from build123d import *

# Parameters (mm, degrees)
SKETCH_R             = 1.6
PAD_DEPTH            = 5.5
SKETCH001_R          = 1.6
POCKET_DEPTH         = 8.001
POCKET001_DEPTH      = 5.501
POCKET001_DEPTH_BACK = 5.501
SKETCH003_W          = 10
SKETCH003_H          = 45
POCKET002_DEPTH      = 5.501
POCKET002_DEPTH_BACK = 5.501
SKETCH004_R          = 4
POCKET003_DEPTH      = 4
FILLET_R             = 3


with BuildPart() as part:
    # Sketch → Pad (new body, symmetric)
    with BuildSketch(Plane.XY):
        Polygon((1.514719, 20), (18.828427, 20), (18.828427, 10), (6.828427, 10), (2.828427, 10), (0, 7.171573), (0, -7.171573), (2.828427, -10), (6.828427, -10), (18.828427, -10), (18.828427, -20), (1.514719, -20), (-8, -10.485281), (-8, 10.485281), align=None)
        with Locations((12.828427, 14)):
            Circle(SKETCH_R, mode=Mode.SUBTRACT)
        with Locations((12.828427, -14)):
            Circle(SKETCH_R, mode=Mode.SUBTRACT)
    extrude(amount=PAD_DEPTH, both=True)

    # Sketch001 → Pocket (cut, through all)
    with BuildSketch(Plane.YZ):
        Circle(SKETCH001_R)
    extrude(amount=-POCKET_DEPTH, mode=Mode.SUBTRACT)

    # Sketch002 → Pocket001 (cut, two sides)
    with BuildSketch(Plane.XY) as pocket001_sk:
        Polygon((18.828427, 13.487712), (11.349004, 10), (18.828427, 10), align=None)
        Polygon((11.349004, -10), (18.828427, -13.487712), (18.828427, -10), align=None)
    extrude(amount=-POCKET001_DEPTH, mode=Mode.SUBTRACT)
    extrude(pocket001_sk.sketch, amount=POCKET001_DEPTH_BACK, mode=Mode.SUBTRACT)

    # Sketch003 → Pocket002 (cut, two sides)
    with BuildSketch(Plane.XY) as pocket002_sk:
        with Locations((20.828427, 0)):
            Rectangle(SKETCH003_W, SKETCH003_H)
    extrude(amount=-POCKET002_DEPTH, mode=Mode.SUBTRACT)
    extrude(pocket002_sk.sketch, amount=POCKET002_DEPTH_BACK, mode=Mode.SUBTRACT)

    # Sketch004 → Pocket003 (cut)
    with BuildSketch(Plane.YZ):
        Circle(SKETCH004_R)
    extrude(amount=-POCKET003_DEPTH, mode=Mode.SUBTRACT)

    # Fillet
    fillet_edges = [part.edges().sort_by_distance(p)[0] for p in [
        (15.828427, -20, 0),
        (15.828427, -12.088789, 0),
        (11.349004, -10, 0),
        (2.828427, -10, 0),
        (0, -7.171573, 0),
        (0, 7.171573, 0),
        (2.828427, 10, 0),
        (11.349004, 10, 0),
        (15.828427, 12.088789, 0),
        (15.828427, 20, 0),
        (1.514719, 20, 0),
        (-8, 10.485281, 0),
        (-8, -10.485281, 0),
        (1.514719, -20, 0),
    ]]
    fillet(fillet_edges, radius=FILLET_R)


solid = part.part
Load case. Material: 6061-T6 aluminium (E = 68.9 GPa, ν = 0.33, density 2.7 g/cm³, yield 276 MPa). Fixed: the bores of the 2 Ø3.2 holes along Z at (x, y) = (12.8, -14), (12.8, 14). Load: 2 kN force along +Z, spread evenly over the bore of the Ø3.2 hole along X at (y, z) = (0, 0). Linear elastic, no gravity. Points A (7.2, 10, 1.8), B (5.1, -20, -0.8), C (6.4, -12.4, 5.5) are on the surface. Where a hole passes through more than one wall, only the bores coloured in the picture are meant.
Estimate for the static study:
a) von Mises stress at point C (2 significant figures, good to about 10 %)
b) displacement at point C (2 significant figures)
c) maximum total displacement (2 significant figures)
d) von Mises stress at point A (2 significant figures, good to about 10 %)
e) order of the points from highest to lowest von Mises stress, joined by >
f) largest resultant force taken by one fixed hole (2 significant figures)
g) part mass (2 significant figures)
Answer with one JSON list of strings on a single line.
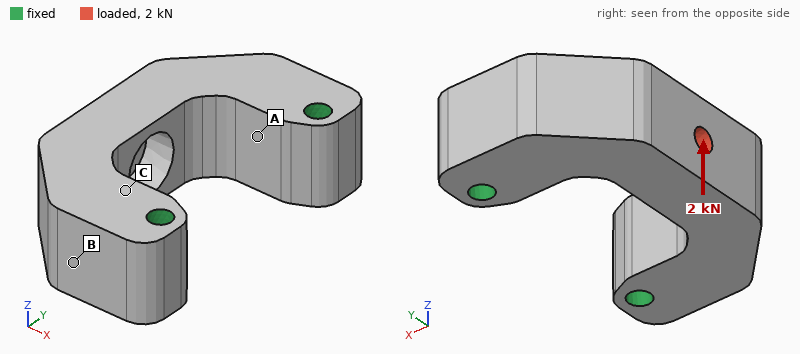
["85 MPa", "13 µm", "68 µm", "58 MPa", "C > A > B", "1.0 kN", "15 g"]
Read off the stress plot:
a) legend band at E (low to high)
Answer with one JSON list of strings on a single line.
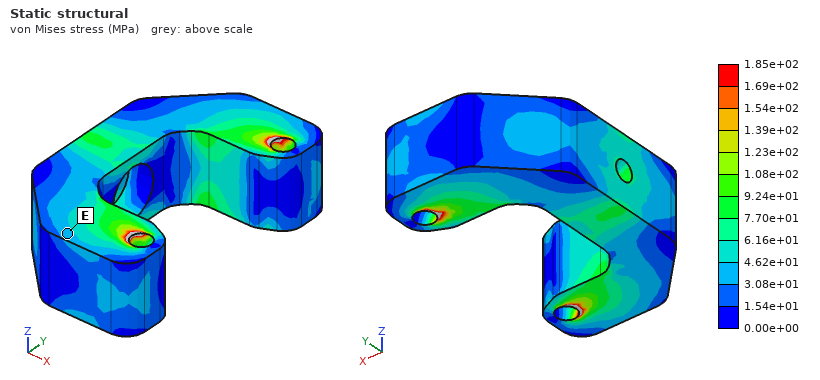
["3.08e+01 to 4.62e+01 MPa"]
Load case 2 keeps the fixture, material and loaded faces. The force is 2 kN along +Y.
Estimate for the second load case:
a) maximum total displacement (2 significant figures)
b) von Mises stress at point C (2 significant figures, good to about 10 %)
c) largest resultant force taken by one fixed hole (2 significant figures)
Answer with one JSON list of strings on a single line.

["26 µm", "26 MPa", "1.3 kN"]
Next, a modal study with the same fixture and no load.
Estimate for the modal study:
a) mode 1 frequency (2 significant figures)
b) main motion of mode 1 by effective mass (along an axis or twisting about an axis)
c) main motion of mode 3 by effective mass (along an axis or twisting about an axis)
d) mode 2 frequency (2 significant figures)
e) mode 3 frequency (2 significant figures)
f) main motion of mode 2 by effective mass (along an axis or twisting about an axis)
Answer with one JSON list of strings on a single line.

["14 kHz", "along Z", "twisting about X", "17 kHz", "26 kHz", "along Y"]
